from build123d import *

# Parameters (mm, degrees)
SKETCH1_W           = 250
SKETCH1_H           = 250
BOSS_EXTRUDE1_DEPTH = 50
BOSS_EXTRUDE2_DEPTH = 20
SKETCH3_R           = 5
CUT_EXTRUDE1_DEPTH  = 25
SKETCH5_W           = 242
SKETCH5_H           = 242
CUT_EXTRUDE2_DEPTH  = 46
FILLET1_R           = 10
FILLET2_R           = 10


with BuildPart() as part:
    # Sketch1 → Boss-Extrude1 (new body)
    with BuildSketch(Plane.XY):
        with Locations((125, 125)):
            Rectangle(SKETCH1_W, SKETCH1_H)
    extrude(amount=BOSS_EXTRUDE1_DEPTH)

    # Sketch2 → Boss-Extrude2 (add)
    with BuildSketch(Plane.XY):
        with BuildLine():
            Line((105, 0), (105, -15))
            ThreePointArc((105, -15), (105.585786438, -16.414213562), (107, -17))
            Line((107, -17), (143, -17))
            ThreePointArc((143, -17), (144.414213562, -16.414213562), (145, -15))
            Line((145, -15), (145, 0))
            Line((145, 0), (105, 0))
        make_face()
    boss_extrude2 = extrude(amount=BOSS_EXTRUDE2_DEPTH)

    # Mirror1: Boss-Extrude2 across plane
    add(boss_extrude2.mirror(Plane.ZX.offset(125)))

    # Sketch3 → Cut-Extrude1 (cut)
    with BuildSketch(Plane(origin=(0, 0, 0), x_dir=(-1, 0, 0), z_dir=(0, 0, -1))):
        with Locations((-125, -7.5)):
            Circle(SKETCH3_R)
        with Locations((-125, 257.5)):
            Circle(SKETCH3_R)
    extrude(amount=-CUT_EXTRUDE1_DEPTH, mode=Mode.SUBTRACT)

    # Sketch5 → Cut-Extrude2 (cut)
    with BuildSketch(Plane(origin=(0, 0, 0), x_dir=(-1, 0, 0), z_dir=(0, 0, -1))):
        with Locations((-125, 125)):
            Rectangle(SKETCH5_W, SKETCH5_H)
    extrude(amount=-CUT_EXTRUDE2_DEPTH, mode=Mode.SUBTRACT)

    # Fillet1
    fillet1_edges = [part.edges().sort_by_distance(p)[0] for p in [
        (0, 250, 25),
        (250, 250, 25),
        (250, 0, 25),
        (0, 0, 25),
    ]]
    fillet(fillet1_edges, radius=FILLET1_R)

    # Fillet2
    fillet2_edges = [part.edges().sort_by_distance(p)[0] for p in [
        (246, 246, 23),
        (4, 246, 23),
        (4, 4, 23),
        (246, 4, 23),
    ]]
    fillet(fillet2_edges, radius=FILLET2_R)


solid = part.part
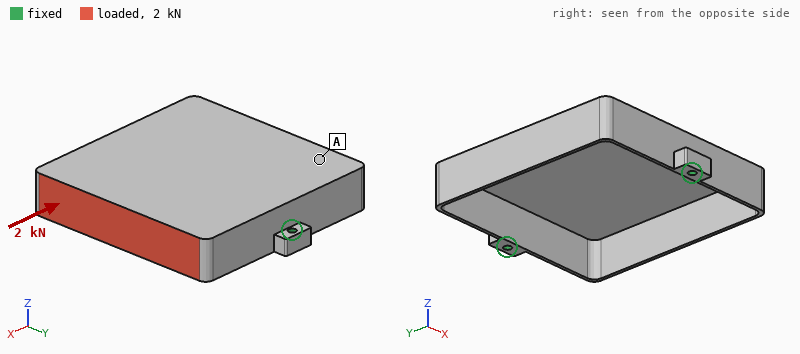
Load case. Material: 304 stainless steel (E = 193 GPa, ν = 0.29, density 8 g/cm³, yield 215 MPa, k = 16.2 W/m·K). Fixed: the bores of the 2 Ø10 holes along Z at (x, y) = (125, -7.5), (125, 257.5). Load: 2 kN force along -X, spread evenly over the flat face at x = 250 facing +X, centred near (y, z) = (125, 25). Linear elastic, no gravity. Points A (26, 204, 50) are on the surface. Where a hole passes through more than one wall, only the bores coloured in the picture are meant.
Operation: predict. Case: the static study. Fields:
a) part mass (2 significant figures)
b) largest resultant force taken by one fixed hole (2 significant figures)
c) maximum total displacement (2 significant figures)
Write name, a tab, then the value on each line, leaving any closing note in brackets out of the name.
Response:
part mass	3.6 kg
largest resultant force taken by one fixed hole	1.0 kN
maximum total displacement	0.26 mm
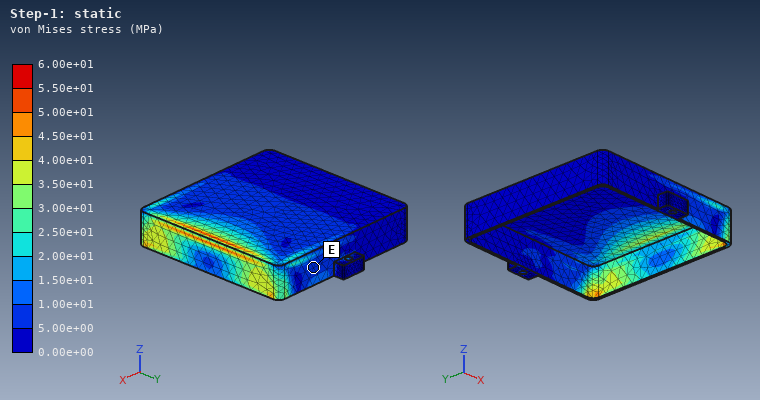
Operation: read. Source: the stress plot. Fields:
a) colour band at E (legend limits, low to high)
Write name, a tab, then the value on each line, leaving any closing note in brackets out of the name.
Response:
colour band at E	5.00e+00 to 1.00e+01 MPa
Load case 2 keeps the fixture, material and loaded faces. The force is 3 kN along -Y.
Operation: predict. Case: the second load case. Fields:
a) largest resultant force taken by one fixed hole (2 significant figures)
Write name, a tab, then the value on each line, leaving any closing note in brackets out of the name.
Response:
largest resultant force taken by one fixed hole	2.1 kN
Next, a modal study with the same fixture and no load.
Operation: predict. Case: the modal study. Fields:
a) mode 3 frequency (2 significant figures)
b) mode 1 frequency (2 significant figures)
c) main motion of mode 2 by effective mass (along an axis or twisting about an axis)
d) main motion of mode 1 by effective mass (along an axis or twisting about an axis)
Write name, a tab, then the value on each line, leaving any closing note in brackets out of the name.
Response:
mode 3 frequency	560 Hz
mode 1 frequency	430 Hz
main motion of mode 2 by effective mass	along Y
main motion of mode 1 by effective mass	along Z
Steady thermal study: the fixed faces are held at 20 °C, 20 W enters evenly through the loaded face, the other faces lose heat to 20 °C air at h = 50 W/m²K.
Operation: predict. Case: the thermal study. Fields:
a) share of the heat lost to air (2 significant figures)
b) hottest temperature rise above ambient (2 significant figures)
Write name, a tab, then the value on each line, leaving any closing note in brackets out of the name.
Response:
share of the heat lost to air	100 %
hottest temperature rise above ambient	22 K
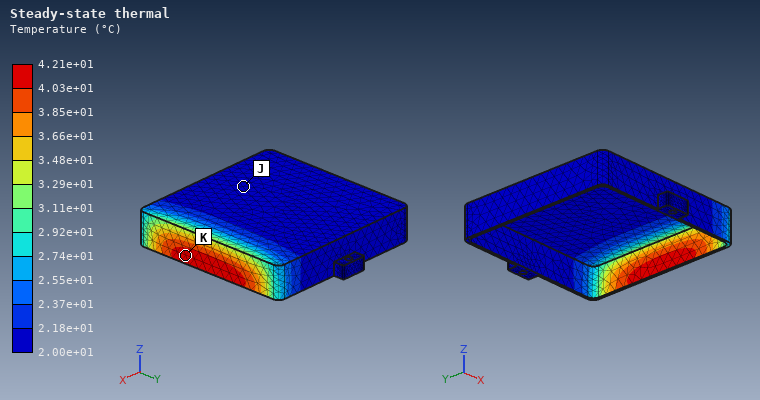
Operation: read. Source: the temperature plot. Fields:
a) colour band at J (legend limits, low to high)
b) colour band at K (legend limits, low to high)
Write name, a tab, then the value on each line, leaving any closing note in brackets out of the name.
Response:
colour band at J	2.00e+01 to 2.18e+01 °C
colour band at K	4.03e+01 to 4.21e+01 °C
